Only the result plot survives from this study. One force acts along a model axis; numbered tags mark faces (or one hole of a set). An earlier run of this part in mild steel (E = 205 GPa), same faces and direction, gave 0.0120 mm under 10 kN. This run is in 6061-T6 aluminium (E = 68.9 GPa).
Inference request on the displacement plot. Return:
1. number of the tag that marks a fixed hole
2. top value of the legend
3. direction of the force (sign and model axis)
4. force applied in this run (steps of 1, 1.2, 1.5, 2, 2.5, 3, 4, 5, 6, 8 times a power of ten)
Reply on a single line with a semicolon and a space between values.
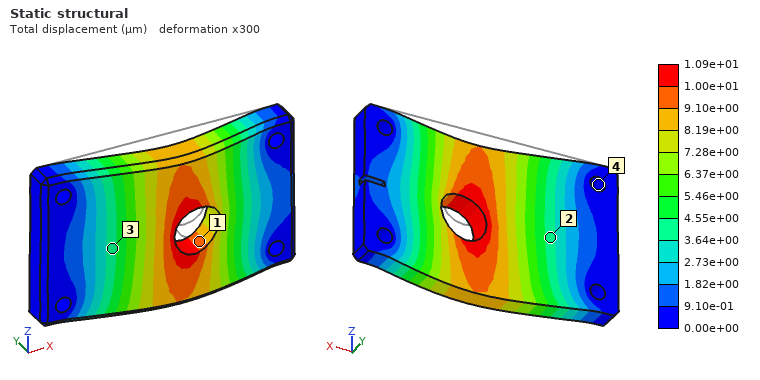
4; 1.09e+01 µm; -Z; 3 kN
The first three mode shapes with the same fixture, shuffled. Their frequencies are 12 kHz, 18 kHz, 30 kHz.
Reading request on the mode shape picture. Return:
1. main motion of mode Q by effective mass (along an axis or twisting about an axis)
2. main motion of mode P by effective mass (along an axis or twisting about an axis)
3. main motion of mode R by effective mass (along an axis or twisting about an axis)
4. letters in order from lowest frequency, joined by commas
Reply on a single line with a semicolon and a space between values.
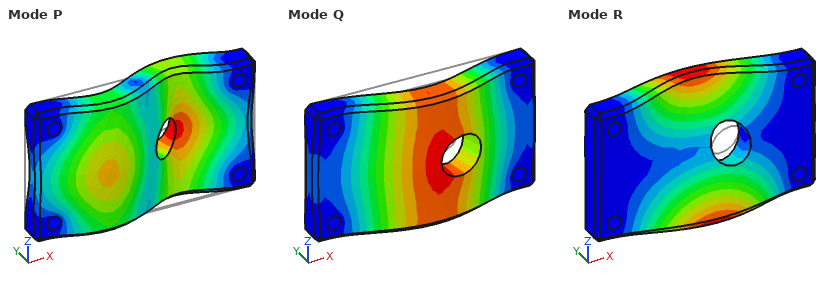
along Y; twisting about Z; twisting about X; Q, R, P
